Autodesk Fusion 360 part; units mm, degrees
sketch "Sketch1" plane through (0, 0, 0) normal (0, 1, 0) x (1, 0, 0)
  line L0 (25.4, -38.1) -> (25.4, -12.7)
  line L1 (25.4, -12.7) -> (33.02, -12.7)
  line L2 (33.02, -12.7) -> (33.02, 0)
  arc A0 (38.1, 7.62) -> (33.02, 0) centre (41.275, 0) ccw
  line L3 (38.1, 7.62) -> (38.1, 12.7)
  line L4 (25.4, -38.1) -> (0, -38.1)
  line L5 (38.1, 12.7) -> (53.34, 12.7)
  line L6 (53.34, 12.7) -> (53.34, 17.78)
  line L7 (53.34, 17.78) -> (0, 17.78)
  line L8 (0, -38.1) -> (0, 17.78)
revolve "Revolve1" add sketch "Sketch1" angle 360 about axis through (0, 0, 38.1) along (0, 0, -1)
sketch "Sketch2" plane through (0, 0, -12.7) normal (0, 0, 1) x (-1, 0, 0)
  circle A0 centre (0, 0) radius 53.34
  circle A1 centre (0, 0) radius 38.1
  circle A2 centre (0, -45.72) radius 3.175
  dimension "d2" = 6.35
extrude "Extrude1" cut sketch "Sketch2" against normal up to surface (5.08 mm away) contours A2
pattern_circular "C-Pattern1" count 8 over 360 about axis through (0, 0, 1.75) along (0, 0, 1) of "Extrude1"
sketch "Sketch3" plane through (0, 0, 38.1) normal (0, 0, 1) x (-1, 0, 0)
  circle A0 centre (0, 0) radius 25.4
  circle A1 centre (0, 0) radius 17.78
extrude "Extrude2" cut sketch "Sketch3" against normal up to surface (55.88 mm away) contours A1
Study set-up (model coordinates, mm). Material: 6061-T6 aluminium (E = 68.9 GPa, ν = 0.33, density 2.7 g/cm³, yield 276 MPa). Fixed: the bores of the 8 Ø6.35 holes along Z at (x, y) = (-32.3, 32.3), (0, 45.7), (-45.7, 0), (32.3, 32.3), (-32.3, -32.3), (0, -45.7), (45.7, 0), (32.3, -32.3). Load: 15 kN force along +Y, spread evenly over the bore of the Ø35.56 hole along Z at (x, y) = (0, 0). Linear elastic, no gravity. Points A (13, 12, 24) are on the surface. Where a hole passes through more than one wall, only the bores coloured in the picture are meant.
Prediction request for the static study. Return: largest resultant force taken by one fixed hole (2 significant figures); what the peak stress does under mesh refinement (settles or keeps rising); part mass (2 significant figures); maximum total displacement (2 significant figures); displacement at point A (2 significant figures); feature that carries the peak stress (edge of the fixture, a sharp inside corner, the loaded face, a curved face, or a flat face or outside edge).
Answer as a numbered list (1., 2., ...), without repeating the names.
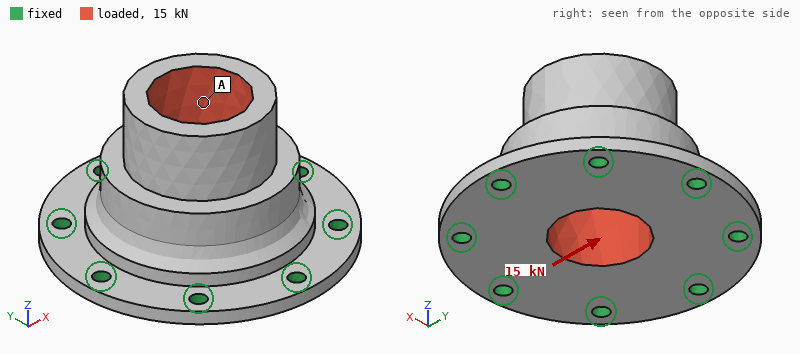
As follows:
1. 3.6 kN
2. keeps rising
3. 370 g
4. 42 µm
5. 30 µm
6. edge of the fixture
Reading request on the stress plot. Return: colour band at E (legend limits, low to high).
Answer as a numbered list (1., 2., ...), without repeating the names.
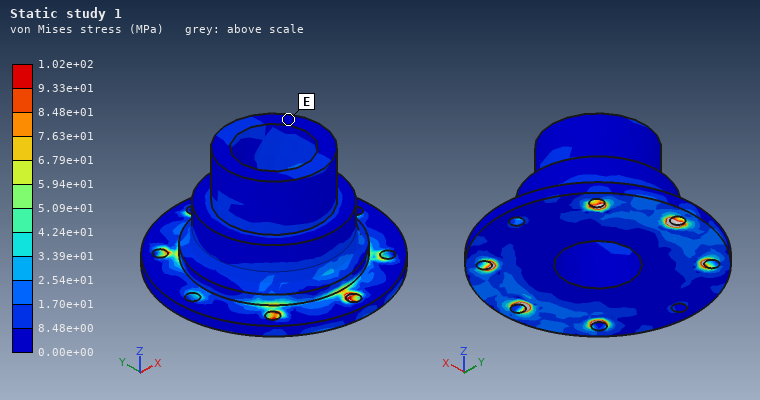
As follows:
1. 0.00e+00 to 8.48e+00 MPa
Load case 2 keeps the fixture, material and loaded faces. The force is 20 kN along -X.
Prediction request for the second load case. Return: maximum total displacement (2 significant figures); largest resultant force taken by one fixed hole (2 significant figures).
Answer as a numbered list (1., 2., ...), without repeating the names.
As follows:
1. 56 µm
2. 4.8 kN
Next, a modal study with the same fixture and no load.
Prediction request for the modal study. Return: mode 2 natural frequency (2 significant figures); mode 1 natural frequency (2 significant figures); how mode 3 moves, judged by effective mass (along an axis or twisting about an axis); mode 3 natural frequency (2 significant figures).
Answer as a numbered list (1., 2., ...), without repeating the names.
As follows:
1. 7700 Hz
2. 7700 Hz
3. along Z
4. 8400 Hz
